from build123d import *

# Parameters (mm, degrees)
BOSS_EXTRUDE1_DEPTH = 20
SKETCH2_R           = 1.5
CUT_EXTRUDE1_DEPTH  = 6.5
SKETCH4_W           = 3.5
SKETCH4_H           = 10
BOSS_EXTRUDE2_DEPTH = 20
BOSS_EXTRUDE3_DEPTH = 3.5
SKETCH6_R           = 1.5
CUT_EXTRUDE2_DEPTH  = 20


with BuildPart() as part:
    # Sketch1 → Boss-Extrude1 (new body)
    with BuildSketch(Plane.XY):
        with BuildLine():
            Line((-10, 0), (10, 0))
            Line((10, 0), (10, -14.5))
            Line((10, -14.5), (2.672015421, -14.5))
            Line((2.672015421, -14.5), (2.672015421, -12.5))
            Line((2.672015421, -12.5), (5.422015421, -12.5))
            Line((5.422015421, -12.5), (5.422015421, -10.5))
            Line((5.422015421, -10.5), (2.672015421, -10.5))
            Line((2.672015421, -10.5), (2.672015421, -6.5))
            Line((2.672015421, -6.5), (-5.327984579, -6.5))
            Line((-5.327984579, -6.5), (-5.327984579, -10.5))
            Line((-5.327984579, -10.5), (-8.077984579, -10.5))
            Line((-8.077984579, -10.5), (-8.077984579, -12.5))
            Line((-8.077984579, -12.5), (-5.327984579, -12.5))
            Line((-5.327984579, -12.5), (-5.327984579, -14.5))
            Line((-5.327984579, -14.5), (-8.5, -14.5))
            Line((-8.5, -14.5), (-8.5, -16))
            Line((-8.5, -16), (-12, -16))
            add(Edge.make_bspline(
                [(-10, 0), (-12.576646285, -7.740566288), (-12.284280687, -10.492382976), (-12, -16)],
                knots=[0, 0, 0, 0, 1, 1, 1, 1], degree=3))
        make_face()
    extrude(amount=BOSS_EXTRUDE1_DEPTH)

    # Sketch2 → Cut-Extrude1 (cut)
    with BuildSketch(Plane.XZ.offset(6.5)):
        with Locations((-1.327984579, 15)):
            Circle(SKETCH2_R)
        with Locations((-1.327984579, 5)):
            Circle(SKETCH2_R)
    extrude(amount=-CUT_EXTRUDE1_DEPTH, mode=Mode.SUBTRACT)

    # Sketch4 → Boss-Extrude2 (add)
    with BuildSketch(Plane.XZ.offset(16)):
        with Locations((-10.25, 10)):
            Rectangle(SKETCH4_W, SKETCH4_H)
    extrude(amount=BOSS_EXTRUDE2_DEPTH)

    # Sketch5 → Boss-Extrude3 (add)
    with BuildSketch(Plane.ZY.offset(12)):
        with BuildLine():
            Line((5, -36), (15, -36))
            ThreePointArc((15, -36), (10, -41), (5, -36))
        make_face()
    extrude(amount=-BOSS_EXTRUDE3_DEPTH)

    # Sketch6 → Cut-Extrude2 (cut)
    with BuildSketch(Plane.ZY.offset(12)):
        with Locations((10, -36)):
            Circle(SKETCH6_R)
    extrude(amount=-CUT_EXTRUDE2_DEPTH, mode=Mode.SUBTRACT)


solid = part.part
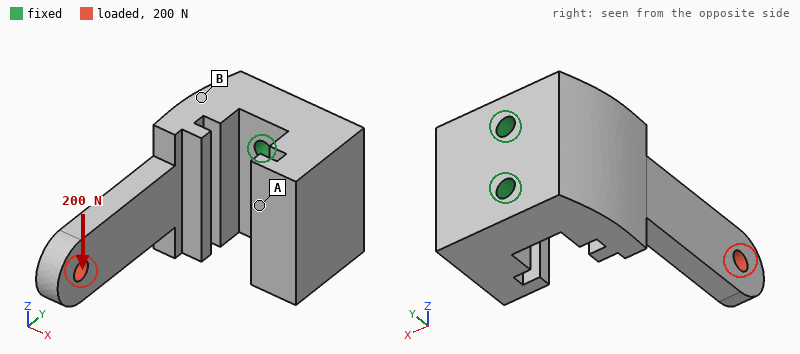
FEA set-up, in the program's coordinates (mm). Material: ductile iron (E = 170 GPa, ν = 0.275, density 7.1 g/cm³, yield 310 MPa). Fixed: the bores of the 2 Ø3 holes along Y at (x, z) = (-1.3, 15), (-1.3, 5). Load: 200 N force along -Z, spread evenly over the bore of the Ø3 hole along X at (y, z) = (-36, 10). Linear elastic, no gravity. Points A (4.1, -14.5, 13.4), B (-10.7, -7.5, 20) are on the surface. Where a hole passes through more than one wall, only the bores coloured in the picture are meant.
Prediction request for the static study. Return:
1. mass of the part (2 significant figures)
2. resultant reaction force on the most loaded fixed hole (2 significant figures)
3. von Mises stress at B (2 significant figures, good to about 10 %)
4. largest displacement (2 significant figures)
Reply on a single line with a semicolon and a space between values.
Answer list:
40 g; 470 N; 14 MPa; 35 µm
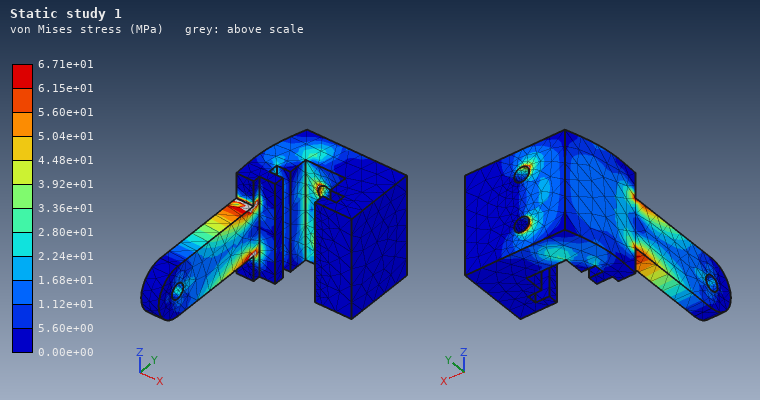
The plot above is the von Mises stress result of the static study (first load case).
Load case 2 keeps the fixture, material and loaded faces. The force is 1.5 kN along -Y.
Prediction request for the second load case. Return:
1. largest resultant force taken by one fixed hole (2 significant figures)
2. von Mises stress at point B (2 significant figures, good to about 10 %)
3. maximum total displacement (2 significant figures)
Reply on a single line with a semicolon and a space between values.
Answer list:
750 N; 18 MPa; 41 µm
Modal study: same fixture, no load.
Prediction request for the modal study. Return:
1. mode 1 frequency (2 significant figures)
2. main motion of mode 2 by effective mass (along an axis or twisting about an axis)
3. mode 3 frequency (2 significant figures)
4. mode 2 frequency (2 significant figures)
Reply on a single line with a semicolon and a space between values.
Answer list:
3300 Hz; along Z; 13 kHz; 7900 Hz
